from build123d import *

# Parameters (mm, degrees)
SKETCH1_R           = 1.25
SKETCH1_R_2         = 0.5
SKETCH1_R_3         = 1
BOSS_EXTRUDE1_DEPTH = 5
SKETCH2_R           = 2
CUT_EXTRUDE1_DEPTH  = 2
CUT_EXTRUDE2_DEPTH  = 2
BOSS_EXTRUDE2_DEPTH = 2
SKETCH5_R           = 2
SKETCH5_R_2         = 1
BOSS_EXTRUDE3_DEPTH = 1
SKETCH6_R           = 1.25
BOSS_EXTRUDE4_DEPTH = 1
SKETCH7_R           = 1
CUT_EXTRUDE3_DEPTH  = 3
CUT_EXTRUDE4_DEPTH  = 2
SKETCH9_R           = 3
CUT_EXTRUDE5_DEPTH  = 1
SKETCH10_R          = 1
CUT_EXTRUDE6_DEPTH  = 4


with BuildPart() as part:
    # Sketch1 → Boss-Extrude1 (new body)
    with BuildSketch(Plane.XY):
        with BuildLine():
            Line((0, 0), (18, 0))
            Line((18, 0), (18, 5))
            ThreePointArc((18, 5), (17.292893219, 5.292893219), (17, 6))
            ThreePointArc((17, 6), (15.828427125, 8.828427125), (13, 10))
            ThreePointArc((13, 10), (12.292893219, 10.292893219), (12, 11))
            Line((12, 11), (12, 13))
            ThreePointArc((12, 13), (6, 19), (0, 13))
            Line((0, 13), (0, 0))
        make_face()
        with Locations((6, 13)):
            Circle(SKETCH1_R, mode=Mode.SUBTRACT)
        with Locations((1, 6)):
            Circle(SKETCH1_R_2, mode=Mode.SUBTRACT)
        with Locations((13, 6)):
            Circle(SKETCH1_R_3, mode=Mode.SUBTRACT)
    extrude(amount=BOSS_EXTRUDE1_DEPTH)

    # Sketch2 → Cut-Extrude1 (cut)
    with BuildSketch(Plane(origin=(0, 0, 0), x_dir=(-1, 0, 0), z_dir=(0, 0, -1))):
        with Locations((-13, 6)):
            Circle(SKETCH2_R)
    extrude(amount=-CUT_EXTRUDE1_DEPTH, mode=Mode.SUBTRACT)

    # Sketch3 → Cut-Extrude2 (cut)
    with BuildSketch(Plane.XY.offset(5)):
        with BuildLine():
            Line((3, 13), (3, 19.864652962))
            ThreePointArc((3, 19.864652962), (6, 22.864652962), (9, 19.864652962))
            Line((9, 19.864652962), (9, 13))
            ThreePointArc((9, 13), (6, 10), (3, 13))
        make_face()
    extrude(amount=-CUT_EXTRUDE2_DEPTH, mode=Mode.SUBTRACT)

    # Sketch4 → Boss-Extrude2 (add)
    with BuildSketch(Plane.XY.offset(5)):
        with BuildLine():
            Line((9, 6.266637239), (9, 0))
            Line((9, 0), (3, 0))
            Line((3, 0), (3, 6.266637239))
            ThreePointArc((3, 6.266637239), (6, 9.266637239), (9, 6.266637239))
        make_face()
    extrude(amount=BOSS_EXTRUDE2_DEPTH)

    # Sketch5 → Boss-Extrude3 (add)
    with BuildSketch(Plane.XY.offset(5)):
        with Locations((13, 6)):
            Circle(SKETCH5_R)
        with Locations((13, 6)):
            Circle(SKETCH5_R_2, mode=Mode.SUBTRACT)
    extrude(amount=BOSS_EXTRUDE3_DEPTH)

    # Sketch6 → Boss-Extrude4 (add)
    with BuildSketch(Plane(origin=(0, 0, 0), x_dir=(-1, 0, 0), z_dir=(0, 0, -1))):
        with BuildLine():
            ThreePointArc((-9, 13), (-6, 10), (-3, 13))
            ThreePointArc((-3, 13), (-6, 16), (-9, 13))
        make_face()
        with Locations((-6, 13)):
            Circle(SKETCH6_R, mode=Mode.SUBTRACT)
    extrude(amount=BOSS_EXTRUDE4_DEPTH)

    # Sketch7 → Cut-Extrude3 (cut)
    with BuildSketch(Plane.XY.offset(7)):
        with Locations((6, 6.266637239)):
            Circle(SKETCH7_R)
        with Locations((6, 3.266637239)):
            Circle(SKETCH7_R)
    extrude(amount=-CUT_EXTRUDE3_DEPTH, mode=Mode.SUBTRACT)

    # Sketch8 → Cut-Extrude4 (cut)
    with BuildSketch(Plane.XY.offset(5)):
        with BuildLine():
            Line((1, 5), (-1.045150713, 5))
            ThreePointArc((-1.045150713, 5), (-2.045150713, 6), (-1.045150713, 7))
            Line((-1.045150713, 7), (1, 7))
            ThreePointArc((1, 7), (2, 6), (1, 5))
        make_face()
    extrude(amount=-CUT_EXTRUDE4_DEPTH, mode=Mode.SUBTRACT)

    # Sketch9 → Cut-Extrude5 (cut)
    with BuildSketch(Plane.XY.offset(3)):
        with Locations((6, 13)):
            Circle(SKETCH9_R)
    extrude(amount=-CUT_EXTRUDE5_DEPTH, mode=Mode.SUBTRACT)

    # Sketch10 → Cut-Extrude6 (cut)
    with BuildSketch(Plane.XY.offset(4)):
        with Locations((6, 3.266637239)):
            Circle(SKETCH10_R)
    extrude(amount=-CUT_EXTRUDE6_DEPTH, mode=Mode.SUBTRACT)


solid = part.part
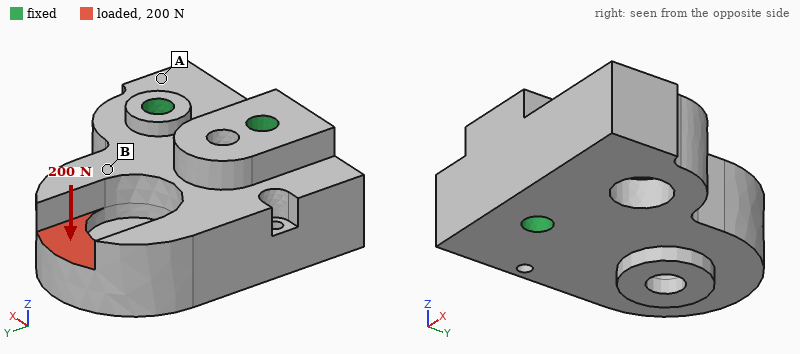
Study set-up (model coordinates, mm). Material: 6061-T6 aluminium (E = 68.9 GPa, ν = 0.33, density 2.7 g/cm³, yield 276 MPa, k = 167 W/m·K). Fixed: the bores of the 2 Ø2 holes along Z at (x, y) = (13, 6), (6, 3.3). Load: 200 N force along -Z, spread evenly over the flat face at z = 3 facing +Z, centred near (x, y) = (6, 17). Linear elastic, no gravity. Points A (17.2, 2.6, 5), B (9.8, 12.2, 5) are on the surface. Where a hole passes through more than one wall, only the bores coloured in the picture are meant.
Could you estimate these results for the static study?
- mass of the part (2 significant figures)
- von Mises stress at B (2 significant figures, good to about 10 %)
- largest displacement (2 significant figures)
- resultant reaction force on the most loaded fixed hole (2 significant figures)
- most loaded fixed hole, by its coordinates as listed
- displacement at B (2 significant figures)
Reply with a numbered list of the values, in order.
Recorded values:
1. 3.4 g
2. 36 MPa
3. 27 µm
4. 120 N
5. (6, 3.3)
6. 8.6 µm
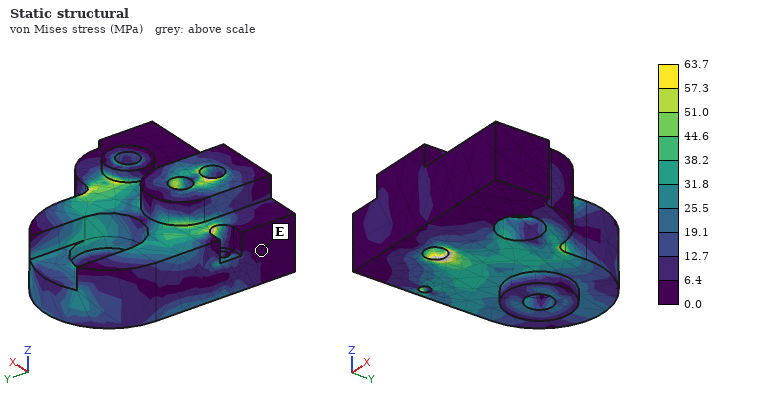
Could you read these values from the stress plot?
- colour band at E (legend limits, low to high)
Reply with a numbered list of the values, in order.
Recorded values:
1. 0.0 to 6.4 MPa
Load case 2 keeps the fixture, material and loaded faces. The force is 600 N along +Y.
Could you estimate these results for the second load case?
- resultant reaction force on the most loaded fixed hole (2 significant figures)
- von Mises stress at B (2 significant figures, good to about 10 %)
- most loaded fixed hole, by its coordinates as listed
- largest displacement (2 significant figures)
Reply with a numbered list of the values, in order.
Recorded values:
1. 520 N
2. 37 MPa
3. (6, 3.3)
4. 18 µm
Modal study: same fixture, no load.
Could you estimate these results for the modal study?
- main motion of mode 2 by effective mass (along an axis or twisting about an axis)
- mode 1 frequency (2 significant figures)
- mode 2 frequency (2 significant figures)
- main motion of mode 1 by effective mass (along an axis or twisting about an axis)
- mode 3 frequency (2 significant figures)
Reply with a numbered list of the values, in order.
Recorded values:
1. along X
2. 22 kHz
3. 35 kHz
4. along Z
5. 46 kHz
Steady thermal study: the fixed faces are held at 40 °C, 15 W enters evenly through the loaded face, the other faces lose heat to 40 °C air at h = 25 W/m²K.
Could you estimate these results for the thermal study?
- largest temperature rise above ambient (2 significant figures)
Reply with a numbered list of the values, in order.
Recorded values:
1. 33 K
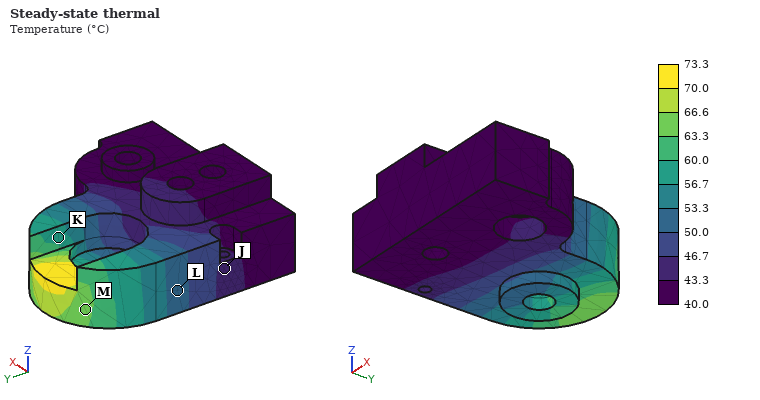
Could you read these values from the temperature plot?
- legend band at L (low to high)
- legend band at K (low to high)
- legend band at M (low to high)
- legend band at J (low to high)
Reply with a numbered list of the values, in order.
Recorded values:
1. 50.0 to 53.3 °C
2. 56.7 to 60.0 °C
3. 63.3 to 66.6 °C
4. 43.3 to 46.7 °C
